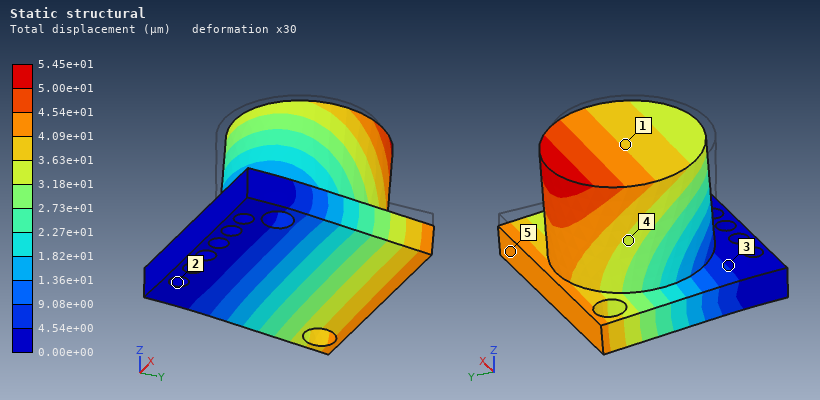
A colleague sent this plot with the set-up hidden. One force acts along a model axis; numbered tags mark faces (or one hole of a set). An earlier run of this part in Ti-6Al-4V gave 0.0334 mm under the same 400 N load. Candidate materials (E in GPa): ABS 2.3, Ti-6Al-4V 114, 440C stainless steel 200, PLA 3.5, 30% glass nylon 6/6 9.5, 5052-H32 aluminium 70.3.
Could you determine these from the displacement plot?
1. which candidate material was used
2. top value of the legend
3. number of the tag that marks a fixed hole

5052-H32 aluminium
5.45e+01 µm
2
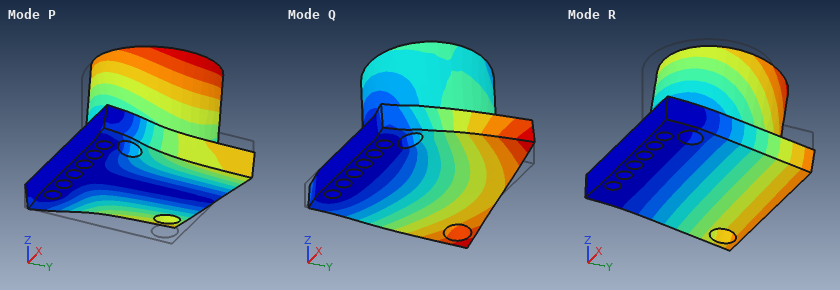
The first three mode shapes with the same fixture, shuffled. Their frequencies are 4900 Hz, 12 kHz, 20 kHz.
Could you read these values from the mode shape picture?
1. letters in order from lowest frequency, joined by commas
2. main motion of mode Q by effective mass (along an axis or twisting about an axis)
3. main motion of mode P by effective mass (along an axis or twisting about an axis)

R, P, Q
along X
along X
